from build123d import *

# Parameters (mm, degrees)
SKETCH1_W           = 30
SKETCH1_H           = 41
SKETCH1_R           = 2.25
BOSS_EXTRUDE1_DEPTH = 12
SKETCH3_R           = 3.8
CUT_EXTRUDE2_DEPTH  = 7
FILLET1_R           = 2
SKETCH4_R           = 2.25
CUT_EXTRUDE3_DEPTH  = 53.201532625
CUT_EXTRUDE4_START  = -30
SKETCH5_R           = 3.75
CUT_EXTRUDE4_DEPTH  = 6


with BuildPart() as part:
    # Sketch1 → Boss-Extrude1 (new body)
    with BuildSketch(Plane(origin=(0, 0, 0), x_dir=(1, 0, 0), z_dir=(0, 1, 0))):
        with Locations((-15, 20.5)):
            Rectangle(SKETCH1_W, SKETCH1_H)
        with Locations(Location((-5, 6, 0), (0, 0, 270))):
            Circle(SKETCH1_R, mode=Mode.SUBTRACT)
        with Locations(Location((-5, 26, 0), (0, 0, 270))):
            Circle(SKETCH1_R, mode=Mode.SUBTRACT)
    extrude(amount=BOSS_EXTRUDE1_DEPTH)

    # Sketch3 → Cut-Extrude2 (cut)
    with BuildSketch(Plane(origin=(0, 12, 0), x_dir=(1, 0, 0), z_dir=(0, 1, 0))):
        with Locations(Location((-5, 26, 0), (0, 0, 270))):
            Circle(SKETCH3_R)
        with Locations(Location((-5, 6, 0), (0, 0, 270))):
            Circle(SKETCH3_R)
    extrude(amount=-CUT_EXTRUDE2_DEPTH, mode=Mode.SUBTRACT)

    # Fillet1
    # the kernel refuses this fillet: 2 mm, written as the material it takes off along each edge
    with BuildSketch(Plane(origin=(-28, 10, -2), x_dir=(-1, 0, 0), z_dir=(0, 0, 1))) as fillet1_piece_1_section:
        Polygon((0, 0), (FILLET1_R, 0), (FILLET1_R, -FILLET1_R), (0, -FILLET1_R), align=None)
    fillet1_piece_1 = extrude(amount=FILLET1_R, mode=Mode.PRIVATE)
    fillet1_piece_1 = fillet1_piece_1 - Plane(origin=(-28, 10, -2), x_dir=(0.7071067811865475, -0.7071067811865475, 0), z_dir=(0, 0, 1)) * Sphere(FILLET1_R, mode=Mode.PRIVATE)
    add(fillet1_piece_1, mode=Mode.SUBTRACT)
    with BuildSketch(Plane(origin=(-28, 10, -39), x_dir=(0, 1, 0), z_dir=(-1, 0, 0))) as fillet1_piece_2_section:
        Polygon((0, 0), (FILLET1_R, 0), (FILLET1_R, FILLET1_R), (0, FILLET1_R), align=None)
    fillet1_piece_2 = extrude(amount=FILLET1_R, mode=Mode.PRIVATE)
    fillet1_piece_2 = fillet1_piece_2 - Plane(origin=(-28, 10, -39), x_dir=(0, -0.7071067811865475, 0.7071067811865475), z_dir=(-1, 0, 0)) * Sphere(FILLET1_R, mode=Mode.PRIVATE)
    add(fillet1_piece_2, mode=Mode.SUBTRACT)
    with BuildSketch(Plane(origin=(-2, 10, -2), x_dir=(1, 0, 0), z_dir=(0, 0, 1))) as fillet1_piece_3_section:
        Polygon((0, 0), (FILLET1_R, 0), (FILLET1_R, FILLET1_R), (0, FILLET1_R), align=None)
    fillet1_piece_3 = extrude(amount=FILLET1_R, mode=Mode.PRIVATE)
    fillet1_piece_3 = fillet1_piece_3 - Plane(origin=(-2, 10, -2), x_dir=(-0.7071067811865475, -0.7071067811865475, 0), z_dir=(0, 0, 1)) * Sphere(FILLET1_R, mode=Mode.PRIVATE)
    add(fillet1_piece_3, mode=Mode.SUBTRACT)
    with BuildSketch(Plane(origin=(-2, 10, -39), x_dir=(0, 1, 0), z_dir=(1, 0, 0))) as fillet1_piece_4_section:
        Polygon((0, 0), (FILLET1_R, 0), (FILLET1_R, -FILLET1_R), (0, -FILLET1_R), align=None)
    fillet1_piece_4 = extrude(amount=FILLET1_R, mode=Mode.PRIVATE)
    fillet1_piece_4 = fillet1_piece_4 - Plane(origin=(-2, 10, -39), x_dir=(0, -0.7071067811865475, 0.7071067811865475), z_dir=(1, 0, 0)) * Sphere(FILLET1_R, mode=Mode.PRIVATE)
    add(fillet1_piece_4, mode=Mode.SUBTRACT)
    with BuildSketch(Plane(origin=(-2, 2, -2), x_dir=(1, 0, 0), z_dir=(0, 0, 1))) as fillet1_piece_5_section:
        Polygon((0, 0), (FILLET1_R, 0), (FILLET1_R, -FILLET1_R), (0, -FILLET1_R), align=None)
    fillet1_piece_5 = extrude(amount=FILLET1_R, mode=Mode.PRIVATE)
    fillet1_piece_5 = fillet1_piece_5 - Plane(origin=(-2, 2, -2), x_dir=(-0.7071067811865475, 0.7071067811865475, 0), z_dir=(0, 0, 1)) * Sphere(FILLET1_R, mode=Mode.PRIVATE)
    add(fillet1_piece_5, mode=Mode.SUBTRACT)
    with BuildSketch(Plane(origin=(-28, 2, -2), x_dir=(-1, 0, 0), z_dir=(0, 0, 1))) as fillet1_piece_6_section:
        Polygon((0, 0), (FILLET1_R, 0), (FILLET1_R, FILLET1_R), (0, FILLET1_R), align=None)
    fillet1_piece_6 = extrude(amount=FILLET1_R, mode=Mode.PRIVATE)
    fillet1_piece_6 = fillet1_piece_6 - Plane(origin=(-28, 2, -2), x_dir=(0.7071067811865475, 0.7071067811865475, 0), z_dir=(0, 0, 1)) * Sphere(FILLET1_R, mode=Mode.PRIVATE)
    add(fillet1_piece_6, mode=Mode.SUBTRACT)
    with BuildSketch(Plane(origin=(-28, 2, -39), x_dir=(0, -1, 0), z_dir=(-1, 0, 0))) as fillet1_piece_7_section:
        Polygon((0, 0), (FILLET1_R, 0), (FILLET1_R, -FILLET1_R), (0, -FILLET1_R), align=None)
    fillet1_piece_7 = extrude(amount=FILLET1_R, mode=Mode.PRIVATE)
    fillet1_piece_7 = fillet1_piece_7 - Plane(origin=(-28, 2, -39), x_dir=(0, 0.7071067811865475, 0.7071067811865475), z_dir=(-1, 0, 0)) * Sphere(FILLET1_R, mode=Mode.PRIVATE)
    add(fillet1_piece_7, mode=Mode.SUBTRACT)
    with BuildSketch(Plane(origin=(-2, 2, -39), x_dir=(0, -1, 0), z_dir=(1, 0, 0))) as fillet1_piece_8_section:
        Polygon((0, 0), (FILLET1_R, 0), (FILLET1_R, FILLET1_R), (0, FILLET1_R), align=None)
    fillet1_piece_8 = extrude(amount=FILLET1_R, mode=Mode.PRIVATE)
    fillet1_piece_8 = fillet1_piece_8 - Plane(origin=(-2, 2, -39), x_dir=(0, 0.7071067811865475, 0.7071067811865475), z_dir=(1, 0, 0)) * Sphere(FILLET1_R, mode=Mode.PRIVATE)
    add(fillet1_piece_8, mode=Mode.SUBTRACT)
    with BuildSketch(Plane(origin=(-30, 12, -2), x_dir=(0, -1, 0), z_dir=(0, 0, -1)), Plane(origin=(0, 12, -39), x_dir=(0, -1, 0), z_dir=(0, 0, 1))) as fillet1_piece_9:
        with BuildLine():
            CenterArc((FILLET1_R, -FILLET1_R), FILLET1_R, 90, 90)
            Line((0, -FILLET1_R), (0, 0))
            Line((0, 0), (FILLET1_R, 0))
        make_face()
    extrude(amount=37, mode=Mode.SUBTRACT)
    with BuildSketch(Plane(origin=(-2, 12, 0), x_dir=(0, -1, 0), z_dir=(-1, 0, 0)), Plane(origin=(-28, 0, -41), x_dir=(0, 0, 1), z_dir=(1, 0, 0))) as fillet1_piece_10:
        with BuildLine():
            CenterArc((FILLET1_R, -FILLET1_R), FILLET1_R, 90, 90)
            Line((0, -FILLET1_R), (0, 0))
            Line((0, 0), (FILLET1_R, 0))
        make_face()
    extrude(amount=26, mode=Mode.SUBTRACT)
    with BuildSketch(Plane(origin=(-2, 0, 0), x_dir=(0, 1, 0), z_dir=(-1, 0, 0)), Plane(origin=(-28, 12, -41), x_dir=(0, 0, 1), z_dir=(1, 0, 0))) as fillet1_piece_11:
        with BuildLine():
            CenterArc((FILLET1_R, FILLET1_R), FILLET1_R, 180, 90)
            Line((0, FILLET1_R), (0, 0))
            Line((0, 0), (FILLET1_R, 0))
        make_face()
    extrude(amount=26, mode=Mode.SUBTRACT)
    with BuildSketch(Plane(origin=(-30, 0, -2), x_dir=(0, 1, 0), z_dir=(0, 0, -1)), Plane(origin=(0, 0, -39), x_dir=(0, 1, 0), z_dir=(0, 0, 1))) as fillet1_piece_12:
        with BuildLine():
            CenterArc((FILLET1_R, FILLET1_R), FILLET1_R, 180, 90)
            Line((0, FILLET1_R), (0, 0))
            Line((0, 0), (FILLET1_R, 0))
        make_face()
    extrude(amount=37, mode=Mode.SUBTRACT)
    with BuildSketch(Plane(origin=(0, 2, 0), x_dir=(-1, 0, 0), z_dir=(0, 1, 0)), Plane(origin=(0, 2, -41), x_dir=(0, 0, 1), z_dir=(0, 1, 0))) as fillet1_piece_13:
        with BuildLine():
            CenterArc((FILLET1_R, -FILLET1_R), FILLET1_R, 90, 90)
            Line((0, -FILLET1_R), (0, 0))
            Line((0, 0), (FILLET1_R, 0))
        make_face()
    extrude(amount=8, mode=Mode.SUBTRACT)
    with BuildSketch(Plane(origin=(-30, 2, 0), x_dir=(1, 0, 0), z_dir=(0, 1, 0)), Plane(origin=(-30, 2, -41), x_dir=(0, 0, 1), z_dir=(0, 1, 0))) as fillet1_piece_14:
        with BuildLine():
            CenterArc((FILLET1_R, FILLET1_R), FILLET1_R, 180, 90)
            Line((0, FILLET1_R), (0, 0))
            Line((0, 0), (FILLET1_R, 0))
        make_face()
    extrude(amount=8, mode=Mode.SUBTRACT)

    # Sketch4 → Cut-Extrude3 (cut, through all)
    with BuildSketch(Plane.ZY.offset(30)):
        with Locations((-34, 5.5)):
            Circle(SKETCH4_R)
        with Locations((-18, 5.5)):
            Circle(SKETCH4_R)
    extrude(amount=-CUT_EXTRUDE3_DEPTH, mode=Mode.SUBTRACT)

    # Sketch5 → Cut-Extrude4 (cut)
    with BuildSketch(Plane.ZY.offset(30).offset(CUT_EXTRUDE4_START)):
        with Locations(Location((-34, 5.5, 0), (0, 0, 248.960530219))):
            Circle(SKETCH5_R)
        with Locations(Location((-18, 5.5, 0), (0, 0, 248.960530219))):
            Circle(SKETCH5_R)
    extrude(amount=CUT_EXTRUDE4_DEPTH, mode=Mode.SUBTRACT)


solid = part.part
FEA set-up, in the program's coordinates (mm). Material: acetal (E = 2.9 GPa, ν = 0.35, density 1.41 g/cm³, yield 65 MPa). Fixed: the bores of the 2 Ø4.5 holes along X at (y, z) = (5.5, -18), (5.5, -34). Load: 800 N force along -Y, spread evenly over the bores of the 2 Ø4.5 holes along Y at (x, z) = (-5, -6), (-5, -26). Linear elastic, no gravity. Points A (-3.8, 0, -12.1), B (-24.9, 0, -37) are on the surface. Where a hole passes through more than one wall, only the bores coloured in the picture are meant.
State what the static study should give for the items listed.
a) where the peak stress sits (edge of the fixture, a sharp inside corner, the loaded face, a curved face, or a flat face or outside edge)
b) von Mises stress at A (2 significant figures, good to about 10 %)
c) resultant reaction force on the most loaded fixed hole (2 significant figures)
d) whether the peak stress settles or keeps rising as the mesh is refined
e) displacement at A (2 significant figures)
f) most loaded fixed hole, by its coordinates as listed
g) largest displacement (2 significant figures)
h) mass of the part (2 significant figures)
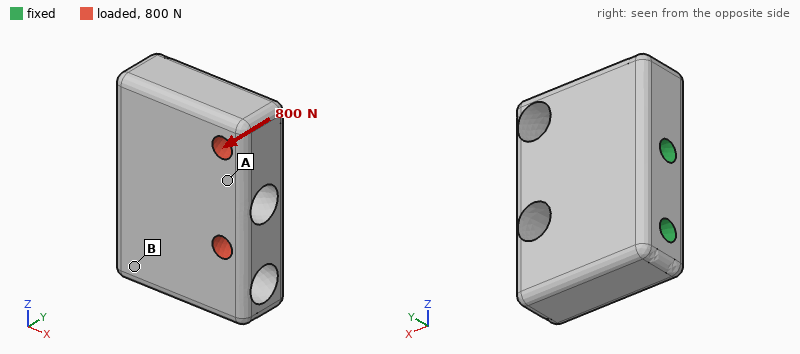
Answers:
edge of the fixture
7.3 MPa
720 N
keeps rising
0.063 mm
(5.5, -18)
0.15 mm
17 g
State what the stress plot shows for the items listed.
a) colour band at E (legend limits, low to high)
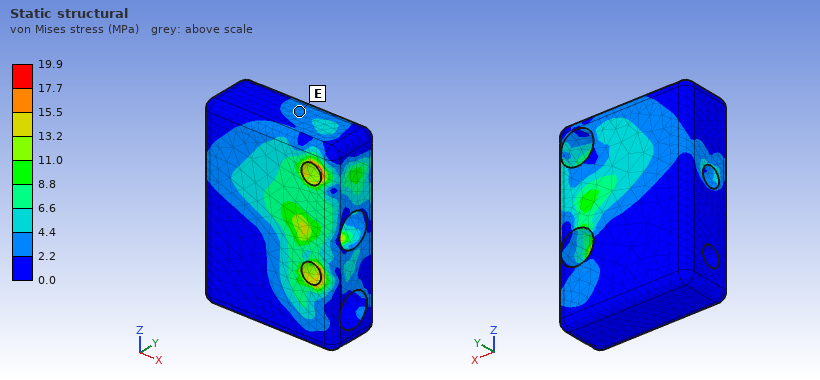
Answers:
2.2 to 4.4 MPa
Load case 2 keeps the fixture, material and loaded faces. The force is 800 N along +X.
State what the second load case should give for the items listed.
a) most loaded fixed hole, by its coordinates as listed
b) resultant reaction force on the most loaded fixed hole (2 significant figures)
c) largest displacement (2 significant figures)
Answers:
(5.5, -18)
630 N
68 µm
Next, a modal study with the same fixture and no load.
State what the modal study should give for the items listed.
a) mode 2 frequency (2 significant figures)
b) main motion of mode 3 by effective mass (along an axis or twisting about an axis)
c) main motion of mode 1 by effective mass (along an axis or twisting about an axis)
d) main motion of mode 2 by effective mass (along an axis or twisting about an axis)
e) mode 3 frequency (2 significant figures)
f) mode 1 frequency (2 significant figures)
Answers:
8600 Hz
along X
along Y
twisting about Z
9000 Hz
5800 Hz
